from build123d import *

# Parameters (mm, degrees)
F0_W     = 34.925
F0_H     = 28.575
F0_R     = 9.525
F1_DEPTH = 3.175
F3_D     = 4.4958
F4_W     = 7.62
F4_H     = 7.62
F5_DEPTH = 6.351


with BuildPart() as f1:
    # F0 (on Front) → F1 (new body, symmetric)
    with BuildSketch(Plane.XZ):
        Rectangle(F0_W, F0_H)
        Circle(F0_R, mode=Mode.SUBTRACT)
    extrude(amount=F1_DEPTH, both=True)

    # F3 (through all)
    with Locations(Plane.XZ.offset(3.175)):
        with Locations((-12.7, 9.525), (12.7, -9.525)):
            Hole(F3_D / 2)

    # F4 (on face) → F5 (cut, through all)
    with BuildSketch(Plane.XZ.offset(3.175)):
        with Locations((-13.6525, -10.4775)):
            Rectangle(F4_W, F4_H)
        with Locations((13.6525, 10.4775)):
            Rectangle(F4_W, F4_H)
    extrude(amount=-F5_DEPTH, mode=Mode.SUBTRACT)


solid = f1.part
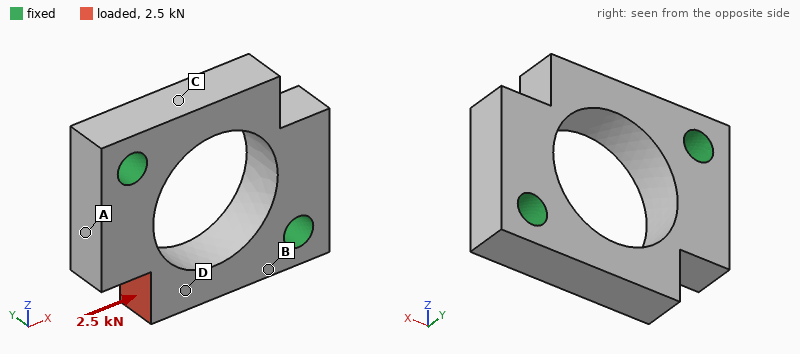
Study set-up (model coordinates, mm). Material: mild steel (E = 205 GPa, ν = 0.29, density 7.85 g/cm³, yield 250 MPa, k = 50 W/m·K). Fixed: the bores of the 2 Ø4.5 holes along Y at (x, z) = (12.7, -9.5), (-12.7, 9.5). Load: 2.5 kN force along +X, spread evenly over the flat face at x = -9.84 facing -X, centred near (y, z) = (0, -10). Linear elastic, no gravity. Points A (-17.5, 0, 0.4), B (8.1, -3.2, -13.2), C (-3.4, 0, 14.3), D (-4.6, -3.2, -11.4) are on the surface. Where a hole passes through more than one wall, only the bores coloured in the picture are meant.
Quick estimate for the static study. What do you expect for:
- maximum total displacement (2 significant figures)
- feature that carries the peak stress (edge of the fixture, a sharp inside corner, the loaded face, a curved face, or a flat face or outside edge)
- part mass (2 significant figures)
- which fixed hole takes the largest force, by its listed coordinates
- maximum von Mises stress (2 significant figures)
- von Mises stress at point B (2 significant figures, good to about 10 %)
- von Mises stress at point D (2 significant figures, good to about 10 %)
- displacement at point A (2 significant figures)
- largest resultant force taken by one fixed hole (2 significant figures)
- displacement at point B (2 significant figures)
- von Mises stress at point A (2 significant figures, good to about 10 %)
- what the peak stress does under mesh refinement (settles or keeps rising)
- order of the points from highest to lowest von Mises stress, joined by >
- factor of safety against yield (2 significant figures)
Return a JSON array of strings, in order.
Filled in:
["8.4 µm", "a curved face", "28 g", "(12.7, -9.5)", "140 MPa", "50 MPa", "71 MPa", "3.8 µm", "2.1 kN", "1.6 µm", "28 MPa", "settles", "D > B > A > C", "1.8"]
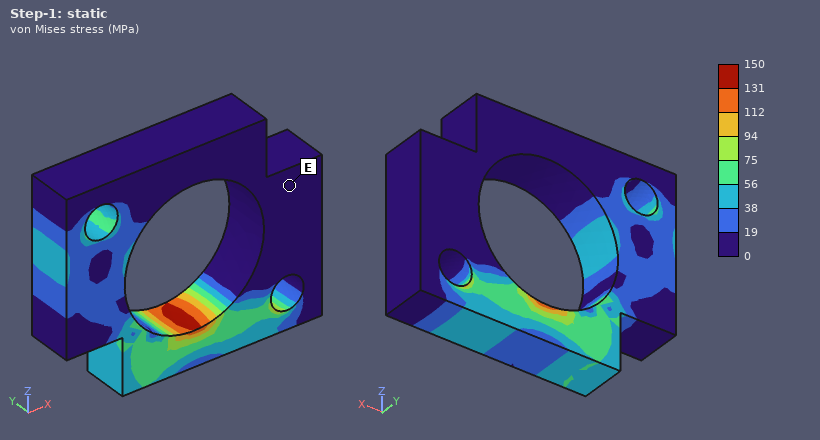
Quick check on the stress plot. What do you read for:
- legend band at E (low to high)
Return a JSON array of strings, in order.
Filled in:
["0 to 19 MPa"]
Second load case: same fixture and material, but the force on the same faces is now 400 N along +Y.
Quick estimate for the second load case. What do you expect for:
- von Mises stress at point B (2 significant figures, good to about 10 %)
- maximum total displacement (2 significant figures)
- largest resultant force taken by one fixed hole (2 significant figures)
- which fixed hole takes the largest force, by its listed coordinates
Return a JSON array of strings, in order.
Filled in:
["43 MPa", "17 µm", "230 N", "(-12.7, 9.5)"]
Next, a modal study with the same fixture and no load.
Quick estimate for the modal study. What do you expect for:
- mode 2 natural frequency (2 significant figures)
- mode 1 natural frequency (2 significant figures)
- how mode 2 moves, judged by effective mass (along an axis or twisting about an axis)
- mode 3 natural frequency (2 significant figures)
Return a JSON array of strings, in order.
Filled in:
["17 kHz", "16 kHz", "along Y", "31 kHz"]
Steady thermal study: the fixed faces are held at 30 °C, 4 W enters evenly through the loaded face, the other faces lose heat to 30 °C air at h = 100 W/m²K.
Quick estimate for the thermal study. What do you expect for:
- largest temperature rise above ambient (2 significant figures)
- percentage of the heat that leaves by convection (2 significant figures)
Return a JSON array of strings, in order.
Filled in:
["22 K", "19 %"]
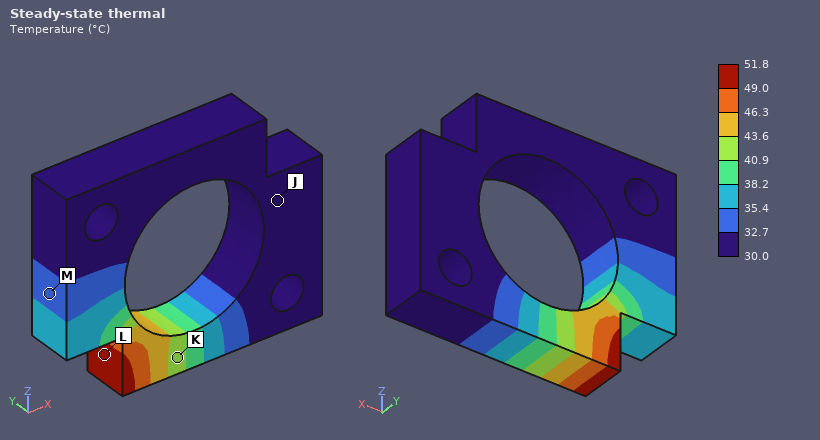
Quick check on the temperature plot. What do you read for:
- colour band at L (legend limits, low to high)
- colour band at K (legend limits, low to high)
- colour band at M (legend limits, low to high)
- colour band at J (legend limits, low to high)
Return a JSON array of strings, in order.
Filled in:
["49.0 to 51.8 °C", "40.9 to 43.6 °C", "32.7 to 35.4 °C", "30.0 to 32.7 °C"]
